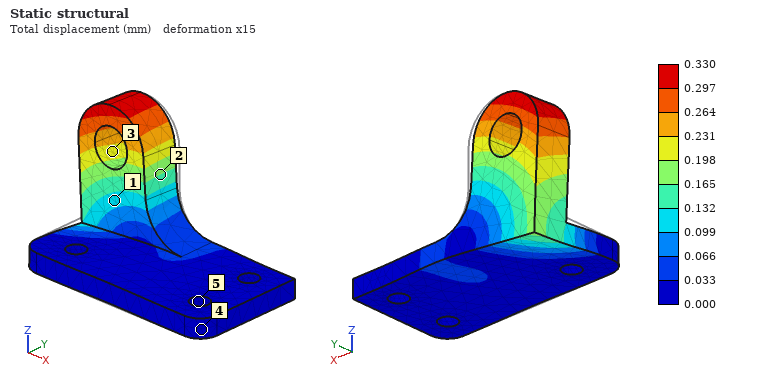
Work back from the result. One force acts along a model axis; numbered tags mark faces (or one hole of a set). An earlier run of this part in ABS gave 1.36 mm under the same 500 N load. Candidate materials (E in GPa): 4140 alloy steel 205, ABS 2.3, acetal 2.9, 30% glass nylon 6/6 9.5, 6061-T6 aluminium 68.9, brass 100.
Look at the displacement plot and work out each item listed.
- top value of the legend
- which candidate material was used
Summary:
0.330 mm
30% glass nylon 6/6
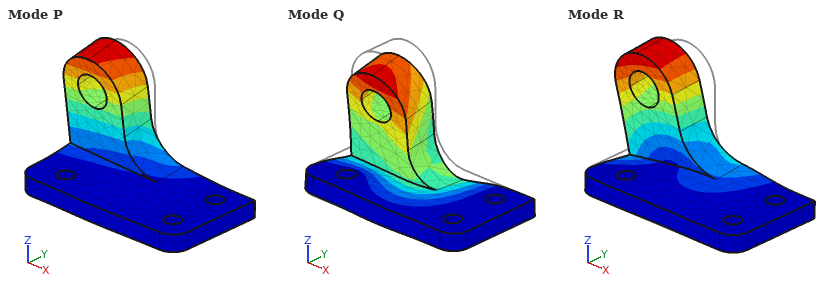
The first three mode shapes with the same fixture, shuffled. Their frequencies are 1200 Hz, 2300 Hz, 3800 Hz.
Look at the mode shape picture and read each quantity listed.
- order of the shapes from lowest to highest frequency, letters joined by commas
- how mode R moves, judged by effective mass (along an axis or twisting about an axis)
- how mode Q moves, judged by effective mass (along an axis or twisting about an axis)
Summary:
P, R, Q
along X
along Z
